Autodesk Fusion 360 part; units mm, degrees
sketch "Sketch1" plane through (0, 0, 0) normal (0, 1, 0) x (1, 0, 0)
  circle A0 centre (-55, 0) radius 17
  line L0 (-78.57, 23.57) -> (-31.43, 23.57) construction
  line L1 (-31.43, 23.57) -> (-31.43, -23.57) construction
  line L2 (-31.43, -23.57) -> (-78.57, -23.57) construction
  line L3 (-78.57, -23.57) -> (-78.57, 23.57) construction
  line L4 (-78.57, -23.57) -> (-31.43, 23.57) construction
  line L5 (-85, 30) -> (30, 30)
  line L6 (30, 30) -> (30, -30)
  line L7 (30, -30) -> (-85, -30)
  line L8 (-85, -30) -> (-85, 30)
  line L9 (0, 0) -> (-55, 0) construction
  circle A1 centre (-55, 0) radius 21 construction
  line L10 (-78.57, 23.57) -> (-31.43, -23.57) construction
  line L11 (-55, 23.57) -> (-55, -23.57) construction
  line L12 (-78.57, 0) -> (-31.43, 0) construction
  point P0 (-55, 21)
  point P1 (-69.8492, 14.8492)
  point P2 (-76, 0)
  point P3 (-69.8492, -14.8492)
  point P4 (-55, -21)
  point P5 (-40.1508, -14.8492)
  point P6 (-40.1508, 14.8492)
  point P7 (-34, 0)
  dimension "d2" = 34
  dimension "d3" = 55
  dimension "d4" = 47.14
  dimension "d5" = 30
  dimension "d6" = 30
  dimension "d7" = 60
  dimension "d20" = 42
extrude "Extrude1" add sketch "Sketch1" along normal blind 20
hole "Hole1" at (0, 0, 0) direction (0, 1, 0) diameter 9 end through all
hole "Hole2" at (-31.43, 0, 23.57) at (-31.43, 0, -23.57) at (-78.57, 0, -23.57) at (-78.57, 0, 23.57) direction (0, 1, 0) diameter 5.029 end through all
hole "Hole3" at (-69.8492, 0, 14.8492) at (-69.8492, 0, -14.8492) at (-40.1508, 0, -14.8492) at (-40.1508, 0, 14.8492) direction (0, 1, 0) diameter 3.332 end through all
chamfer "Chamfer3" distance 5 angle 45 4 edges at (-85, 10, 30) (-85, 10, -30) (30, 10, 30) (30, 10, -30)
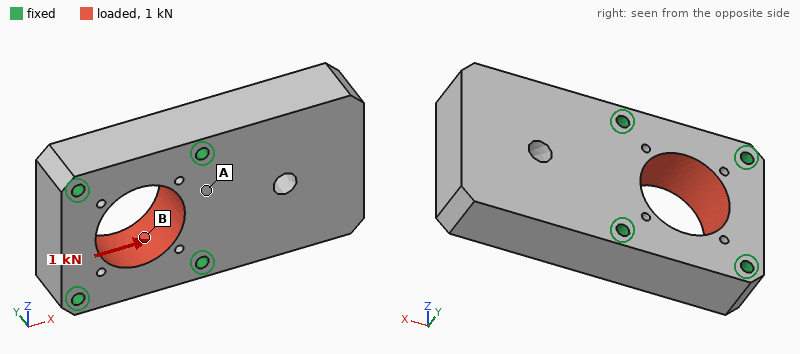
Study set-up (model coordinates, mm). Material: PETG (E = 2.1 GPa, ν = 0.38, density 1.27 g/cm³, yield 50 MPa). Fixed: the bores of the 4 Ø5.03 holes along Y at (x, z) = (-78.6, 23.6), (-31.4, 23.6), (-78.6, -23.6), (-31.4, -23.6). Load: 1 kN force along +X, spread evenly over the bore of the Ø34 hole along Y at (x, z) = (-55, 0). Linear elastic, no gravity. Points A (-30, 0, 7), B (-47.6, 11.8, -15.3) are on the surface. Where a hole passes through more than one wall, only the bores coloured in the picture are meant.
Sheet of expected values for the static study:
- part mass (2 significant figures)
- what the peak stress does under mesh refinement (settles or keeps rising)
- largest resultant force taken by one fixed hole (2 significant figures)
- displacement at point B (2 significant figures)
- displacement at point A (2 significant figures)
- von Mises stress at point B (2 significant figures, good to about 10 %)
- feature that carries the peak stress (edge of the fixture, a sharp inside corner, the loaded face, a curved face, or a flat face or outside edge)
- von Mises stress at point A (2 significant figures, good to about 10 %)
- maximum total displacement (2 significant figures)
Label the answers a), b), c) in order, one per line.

a) 150 g
b) keeps rising
c) 270 N
d) 6.0 µm
e) 5.8 µm
f) 0.88 MPa
g) edge of the fixture
h) 0.35 MPa
i) 21 µm
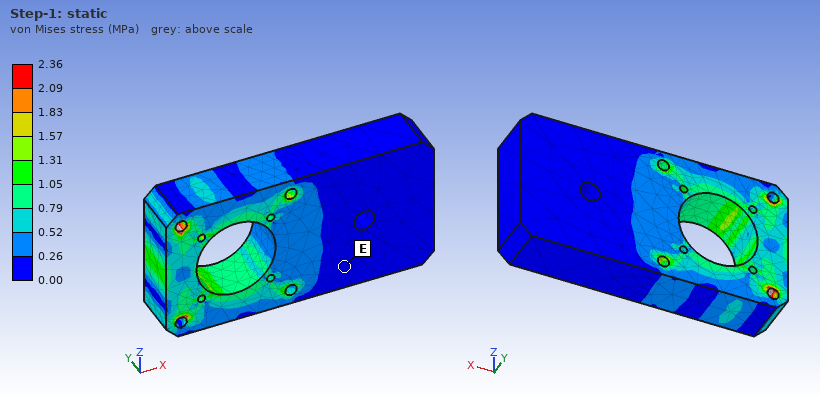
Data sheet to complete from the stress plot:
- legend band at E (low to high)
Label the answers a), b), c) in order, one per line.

a) 0.00 to 0.26 MPa
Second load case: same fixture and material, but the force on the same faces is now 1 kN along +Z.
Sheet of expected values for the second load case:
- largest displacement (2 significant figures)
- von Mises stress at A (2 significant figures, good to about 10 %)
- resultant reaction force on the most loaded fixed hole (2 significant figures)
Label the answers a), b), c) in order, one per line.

a) 19 µm
b) 0.54 MPa
c) 270 N
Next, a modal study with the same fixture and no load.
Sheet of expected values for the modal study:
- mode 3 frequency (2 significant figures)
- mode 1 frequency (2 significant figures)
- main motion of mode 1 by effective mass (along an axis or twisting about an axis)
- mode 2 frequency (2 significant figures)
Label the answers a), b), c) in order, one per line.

a) 2100 Hz
b) 880 Hz
c) along Y
d) 2100 Hz
